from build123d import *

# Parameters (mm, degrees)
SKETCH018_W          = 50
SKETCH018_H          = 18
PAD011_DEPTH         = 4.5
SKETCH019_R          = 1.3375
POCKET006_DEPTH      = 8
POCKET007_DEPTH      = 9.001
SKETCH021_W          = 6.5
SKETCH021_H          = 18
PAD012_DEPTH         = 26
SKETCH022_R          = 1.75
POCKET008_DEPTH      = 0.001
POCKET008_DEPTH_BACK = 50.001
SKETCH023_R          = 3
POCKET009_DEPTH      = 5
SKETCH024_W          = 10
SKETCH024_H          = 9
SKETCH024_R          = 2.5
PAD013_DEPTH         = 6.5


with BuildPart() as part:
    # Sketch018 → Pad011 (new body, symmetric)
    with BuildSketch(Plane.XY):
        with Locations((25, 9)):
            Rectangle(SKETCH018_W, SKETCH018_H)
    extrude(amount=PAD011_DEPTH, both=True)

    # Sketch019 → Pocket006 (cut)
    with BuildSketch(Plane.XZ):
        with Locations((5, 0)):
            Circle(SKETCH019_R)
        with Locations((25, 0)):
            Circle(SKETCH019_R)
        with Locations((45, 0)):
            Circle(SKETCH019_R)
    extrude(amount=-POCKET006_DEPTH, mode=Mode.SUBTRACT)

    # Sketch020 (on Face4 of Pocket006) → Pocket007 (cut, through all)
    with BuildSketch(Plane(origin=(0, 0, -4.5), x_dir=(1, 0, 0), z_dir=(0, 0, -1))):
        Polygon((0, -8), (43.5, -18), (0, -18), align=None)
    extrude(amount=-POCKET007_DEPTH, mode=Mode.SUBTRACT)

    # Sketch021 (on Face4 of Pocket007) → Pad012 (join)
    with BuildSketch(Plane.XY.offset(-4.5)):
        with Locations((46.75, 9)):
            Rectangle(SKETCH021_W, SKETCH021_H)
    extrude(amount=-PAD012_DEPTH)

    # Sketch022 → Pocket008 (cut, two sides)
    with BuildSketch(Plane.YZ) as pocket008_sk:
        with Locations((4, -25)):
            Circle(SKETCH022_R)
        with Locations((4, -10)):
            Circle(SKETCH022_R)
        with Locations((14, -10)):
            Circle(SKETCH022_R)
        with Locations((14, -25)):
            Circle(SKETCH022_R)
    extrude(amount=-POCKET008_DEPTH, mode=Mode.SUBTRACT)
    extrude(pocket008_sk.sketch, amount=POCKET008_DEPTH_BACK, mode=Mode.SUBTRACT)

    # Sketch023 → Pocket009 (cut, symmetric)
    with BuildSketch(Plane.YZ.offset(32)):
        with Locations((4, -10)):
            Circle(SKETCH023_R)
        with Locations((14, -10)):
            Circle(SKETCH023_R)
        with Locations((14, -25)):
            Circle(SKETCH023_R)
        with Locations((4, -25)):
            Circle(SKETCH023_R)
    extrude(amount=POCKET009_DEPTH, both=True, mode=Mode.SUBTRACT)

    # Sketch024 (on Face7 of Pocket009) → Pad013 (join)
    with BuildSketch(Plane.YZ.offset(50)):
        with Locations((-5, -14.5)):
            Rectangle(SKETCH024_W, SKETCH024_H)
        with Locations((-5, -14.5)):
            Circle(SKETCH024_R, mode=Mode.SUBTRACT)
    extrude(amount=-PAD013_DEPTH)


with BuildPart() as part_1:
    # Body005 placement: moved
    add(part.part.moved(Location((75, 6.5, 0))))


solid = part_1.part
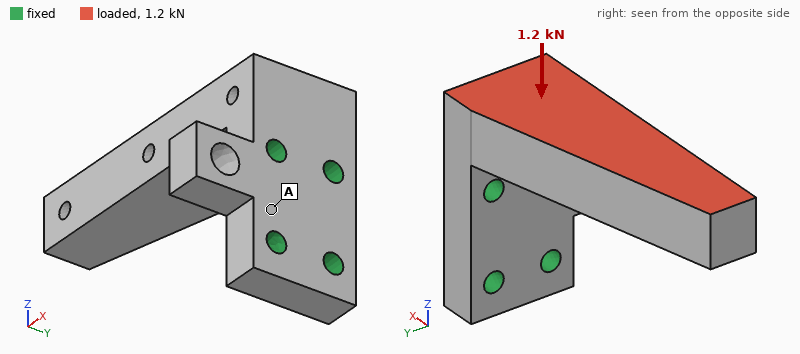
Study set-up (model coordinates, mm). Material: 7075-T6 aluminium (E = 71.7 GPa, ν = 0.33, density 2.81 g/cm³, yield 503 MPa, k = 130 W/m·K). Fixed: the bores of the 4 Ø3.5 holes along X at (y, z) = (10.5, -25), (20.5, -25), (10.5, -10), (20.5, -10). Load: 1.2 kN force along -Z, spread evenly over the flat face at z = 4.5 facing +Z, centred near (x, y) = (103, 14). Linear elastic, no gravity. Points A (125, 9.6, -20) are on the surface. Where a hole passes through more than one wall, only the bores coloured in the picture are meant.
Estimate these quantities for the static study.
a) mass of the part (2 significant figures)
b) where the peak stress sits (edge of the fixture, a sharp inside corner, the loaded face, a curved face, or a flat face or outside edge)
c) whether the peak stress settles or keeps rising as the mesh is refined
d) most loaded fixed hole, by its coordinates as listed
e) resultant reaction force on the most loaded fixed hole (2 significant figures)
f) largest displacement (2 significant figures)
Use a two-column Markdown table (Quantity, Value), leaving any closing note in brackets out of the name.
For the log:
| Quantity | Value |
|---|---|
| mass of the part | 26 g |
| where the peak stress sits | edge of the fixture |
| whether the peak stress settles or keeps rising as the mesh is refined | keeps rising |
| most loaded fixed hole, by its coordinates as listed | (10.5, -10) |
| resultant reaction force on the most loaded fixed hole | 770 N |
| largest displacement | 0.43 mm |
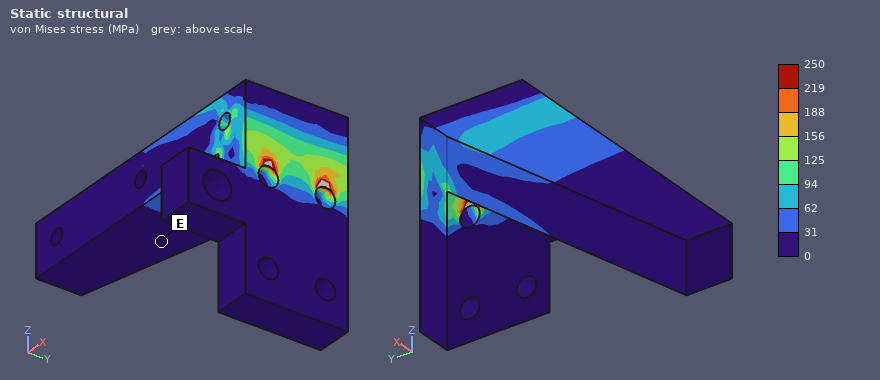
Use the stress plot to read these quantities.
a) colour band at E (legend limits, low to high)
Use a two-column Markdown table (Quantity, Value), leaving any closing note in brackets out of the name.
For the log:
| Quantity | Value |
|---|---|
| colour band at E | 0 to 31 MPa |
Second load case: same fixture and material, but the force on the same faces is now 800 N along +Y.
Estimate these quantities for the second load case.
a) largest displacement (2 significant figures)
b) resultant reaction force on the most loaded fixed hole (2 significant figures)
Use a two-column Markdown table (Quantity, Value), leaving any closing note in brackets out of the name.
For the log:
| Quantity | Value |
|---|---|
| largest displacement | 0.11 mm |
| resultant reaction force on the most loaded fixed hole | 1.4 kN |
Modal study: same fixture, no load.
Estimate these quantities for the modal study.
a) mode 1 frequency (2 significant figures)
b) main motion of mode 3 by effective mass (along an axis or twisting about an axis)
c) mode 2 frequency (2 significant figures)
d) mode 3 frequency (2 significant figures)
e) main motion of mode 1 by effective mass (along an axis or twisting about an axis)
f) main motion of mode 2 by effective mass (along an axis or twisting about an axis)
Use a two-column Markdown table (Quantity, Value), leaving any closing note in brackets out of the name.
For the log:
| Quantity | Value |
|---|---|
| mode 1 frequency | 2600 Hz |
| main motion of mode 3 by effective mass | along X |
| mode 2 frequency | 4200 Hz |
| mode 3 frequency | 13 kHz |
| main motion of mode 1 by effective mass | along Z |
| main motion of mode 2 by effective mass | along Y |
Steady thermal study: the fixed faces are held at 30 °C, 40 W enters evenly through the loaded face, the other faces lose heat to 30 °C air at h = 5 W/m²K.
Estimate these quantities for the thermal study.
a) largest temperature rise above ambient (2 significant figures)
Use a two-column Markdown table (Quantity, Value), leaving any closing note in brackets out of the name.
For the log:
| Quantity | Value |
|---|---|
| largest temperature rise above ambient | 62 K |
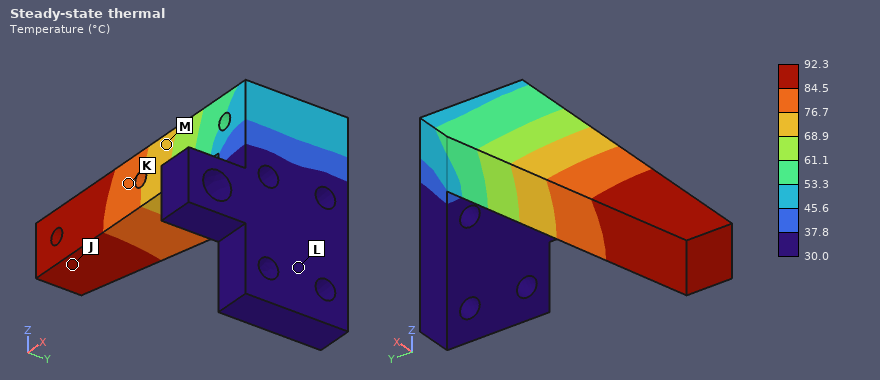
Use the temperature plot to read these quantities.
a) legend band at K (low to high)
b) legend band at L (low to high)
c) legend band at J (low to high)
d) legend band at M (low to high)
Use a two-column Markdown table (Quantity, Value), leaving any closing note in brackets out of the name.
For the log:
| Quantity | Value |
|---|---|
| legend band at K | 76.7 to 84.5 °C |
| legend band at L | 30.0 to 37.8 °C |
| legend band at J | 84.5 to 92.3 °C |
| legend band at M | 68.9 to 76.7 °C |
